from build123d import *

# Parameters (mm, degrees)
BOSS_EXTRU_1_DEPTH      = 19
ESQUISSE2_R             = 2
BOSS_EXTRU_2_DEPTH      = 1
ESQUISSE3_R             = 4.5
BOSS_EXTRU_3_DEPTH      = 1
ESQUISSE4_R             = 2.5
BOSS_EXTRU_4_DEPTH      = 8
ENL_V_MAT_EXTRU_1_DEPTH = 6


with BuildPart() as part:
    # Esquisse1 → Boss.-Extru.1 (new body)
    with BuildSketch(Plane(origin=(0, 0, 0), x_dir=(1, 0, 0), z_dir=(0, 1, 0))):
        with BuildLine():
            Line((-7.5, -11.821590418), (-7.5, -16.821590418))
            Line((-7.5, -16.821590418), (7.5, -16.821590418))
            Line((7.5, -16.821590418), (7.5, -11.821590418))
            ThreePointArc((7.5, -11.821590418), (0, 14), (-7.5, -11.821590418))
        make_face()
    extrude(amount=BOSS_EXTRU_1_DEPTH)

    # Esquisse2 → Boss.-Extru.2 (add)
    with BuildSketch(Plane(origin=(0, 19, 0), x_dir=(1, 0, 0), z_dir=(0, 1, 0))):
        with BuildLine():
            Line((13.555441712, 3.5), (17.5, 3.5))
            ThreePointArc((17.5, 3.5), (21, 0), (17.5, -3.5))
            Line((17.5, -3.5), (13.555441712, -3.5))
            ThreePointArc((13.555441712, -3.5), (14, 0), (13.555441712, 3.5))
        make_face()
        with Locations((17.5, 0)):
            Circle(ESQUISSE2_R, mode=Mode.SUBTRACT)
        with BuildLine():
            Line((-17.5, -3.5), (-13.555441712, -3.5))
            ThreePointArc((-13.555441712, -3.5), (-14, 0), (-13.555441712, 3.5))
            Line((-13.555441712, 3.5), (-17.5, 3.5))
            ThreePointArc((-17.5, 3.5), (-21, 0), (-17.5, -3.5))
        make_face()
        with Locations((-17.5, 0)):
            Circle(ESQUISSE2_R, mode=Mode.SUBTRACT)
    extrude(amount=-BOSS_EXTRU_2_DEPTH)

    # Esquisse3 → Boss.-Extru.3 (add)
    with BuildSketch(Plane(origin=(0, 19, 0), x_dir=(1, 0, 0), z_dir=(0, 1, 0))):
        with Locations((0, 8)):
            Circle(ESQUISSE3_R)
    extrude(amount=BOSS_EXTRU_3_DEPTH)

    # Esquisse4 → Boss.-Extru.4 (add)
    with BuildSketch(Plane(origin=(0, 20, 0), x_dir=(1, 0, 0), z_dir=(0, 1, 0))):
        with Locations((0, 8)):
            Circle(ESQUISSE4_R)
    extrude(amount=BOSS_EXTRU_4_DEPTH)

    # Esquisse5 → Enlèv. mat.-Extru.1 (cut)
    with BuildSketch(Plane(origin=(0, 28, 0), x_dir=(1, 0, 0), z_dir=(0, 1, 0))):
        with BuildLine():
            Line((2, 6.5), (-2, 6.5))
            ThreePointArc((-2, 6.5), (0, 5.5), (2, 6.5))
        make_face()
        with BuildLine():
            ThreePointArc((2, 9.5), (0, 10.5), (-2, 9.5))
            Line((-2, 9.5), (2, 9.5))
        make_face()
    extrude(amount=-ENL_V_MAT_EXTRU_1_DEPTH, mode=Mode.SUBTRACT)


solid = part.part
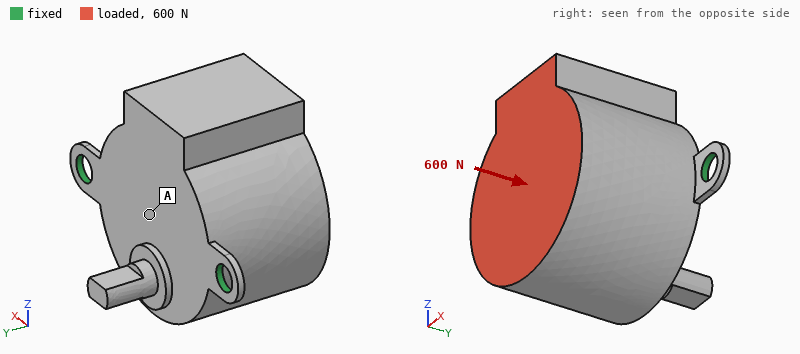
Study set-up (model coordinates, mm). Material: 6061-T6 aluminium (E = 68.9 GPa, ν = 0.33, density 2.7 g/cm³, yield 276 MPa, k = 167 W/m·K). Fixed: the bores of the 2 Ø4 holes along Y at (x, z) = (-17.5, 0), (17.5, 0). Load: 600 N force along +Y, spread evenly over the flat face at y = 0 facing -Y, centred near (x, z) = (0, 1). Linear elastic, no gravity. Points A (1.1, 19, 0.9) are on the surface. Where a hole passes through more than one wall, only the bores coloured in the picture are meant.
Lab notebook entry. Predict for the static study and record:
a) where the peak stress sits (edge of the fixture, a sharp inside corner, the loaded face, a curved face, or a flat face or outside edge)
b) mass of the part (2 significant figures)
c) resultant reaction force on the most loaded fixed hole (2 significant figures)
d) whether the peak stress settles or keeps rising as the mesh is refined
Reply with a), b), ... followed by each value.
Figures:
a) edge of the fixture
b) 35 g
c) 350 N
d) keeps rising
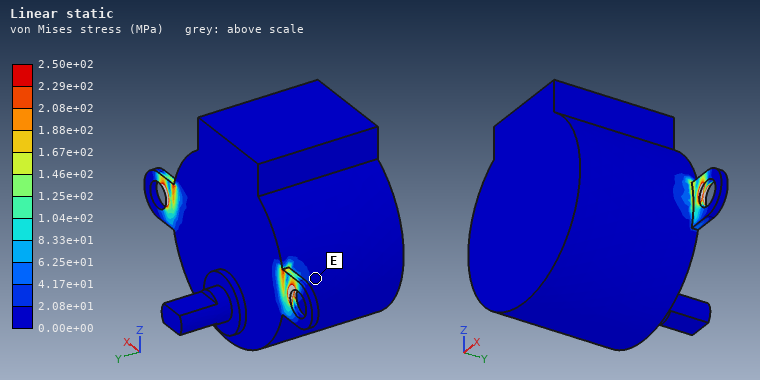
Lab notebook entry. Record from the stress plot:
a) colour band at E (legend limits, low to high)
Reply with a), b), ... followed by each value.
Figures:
a) 0.00e+00 to 2.08e+01 MPa
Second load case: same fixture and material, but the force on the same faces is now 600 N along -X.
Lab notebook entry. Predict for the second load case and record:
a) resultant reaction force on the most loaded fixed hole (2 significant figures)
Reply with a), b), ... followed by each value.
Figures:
a) 480 N
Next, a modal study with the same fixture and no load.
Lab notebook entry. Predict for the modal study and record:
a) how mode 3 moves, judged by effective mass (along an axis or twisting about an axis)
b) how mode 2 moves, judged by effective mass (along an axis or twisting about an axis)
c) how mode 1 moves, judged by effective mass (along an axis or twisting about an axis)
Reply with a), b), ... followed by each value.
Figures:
a) along X
b) along Y
c) along Z
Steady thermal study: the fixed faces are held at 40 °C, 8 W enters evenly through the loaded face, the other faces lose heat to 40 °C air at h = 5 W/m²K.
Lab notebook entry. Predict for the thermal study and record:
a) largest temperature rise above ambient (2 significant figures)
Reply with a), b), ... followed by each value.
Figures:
a) 13 K
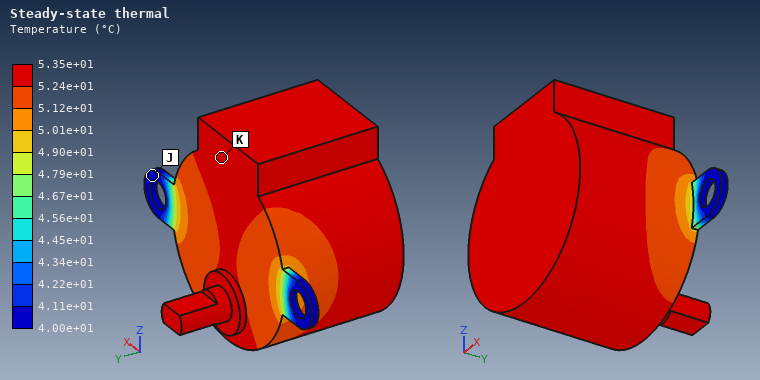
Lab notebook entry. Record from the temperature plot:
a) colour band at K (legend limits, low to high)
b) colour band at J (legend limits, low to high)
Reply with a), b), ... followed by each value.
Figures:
a) 5.24e+01 to 5.35e+01 °C
b) 4.00e+01 to 4.11e+01 °C
